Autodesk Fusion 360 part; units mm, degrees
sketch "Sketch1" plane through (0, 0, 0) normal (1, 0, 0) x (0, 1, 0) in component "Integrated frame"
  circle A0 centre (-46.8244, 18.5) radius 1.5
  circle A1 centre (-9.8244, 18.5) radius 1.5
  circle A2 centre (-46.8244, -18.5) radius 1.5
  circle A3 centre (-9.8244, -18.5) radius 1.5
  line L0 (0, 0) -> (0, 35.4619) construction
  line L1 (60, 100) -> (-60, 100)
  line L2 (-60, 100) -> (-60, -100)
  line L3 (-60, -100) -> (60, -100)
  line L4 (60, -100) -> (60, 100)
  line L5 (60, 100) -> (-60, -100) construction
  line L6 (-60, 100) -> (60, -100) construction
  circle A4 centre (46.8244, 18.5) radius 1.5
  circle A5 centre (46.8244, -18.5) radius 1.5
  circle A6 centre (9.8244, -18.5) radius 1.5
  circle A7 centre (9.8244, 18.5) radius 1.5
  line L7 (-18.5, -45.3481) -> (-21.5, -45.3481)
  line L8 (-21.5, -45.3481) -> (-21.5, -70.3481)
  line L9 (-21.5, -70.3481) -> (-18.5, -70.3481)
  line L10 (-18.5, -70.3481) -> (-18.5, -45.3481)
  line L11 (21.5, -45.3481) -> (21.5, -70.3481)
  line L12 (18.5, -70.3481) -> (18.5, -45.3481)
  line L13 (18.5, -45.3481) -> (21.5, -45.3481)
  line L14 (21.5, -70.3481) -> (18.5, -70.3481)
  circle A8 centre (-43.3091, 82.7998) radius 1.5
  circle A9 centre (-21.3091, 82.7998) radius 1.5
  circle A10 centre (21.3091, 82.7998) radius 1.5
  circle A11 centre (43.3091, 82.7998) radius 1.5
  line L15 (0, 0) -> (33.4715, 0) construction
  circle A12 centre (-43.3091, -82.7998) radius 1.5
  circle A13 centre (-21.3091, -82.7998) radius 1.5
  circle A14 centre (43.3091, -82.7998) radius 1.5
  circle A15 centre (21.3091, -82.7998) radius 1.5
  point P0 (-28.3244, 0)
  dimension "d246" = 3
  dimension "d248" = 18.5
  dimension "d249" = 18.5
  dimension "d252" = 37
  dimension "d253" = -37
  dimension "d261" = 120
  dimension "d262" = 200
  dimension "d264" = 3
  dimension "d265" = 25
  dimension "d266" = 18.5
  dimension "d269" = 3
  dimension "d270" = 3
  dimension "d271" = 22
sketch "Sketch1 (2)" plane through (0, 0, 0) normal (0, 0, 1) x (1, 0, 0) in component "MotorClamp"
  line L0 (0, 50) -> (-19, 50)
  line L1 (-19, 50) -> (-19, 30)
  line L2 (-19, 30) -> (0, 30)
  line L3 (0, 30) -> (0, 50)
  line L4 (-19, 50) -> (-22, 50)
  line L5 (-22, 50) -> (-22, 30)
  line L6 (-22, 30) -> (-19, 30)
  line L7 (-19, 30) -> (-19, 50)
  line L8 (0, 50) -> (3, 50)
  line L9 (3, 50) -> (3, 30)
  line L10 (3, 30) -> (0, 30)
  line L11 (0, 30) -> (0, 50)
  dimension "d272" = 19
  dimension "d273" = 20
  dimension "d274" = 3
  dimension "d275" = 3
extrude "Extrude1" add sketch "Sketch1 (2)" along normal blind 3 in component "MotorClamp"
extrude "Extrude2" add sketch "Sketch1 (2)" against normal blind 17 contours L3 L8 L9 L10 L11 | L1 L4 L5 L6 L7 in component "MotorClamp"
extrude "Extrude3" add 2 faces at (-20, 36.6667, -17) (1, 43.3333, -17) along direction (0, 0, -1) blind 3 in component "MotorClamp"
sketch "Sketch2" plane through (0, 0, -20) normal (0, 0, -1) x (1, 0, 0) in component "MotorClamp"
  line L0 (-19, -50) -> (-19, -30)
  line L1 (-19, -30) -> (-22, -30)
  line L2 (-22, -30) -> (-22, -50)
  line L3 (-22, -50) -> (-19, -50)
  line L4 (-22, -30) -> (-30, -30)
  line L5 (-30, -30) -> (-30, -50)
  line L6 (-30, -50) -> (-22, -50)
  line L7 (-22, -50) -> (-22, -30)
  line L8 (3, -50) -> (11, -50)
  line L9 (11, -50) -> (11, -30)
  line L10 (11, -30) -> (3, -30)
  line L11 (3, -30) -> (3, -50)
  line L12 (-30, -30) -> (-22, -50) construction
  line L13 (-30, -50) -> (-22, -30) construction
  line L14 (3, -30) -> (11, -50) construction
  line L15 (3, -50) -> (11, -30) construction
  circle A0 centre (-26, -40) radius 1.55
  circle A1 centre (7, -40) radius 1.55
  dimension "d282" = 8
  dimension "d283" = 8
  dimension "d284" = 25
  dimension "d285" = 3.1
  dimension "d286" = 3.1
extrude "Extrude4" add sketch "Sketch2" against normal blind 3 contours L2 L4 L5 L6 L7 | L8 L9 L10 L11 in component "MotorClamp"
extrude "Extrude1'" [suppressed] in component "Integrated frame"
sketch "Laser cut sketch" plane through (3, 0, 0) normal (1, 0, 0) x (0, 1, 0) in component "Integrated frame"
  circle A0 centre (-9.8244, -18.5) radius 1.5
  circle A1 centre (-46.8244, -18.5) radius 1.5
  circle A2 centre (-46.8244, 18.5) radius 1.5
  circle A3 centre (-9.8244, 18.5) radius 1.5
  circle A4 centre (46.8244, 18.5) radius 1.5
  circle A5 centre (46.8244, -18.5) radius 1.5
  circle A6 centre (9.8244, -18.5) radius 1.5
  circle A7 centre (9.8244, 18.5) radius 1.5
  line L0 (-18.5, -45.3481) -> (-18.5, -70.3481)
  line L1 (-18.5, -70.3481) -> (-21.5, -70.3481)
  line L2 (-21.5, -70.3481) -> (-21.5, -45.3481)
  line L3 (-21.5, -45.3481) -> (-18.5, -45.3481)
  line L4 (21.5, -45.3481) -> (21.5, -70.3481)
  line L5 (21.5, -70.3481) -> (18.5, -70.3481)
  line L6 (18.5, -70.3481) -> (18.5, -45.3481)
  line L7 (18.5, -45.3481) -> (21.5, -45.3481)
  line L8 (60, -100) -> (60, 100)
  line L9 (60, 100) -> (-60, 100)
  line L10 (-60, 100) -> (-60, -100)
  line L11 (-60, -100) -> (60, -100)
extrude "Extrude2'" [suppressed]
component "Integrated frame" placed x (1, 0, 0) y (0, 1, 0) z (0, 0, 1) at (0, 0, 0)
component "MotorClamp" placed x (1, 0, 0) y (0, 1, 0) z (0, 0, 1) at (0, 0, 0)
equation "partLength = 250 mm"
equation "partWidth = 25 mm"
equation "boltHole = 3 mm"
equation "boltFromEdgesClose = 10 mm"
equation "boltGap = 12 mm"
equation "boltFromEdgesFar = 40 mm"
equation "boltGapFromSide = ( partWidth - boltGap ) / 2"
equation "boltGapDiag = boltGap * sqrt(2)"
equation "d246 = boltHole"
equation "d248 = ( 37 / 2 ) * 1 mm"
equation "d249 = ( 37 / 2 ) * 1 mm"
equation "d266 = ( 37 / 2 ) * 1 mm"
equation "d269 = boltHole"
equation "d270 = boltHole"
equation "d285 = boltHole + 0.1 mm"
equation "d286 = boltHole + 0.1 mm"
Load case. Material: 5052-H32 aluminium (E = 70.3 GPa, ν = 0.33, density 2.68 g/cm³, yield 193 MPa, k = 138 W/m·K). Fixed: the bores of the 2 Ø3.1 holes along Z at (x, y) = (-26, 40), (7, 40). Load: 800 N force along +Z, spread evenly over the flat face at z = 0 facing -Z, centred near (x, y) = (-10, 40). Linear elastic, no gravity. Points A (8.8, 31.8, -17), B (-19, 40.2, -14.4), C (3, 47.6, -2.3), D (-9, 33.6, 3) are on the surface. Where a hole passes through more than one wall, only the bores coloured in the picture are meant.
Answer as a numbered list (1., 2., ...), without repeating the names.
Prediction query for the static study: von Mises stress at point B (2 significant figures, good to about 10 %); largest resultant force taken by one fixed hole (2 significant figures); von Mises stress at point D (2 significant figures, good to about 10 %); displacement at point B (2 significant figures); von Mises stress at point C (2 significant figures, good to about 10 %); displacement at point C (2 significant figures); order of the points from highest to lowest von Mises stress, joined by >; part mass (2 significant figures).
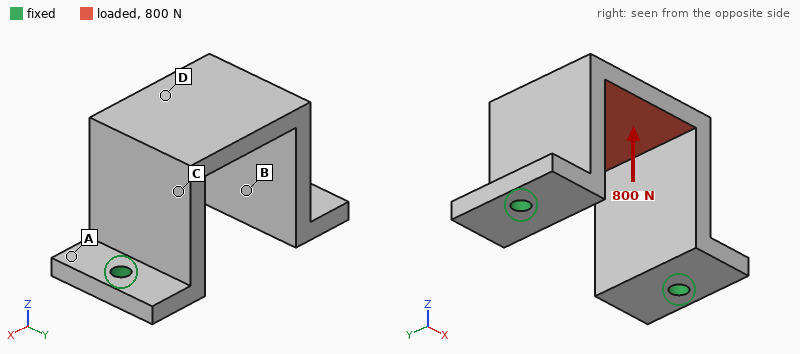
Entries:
1. 11 MPa
2. 420 N
3. 39 MPa
4. 5.4 µm
5. 21 MPa
6. 7.4 µm
7. D > C > B > A
8. 13 g
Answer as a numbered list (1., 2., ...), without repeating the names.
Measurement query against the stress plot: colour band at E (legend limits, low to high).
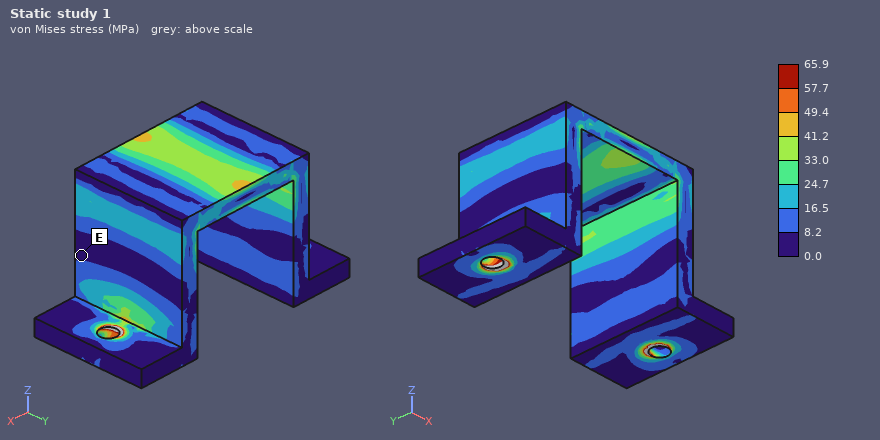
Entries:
1. 0.0 to 8.2 MPa
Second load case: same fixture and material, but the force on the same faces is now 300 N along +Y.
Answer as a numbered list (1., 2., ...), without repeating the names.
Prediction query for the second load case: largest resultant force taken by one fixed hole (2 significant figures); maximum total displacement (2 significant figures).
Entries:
1. 150 N
2. 82 µm
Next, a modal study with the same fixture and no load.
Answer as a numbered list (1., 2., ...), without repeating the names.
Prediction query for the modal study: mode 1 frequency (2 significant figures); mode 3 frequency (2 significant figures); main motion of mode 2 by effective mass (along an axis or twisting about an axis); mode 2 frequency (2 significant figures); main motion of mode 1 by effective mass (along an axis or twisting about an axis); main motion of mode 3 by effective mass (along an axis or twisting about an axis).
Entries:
1. 3900 Hz
2. 7000 Hz
3. along X
4. 4800 Hz
5. along Y
6. twisting about Z
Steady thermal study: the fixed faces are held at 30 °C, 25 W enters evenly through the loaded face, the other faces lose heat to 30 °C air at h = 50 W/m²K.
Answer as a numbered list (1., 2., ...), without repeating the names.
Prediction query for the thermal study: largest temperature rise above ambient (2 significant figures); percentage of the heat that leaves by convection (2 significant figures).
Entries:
1. 43 K
2. 14 %
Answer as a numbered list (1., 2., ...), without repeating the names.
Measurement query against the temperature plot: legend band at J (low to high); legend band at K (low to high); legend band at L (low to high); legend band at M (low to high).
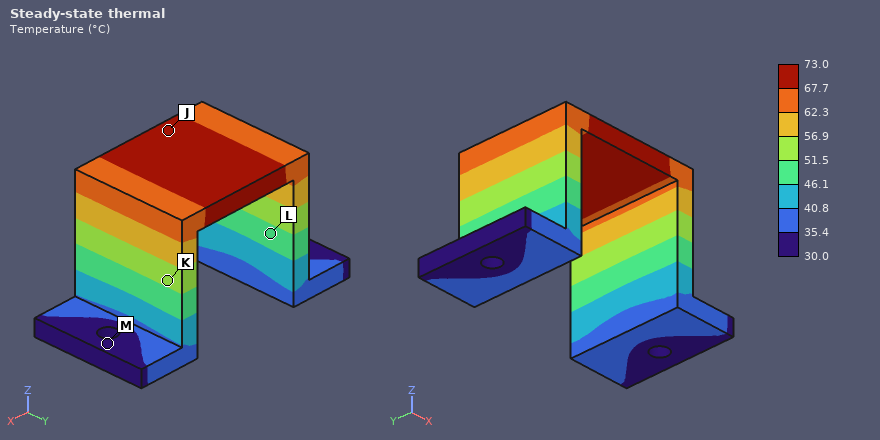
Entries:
1. 67.7 to 73.0 °C
2. 51.5 to 56.9 °C
3. 46.1 to 51.5 °C
4. 30.0 to 35.4 °C
